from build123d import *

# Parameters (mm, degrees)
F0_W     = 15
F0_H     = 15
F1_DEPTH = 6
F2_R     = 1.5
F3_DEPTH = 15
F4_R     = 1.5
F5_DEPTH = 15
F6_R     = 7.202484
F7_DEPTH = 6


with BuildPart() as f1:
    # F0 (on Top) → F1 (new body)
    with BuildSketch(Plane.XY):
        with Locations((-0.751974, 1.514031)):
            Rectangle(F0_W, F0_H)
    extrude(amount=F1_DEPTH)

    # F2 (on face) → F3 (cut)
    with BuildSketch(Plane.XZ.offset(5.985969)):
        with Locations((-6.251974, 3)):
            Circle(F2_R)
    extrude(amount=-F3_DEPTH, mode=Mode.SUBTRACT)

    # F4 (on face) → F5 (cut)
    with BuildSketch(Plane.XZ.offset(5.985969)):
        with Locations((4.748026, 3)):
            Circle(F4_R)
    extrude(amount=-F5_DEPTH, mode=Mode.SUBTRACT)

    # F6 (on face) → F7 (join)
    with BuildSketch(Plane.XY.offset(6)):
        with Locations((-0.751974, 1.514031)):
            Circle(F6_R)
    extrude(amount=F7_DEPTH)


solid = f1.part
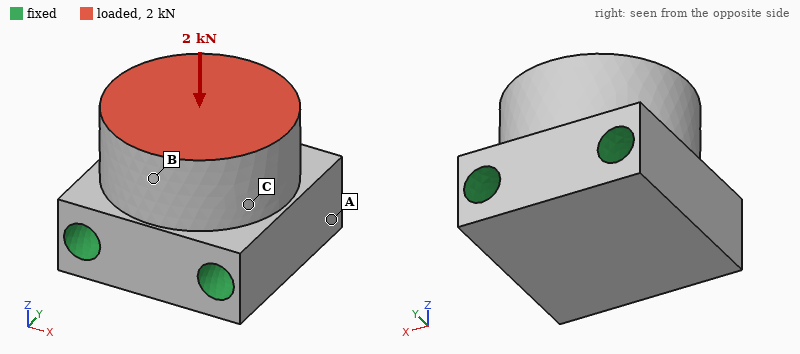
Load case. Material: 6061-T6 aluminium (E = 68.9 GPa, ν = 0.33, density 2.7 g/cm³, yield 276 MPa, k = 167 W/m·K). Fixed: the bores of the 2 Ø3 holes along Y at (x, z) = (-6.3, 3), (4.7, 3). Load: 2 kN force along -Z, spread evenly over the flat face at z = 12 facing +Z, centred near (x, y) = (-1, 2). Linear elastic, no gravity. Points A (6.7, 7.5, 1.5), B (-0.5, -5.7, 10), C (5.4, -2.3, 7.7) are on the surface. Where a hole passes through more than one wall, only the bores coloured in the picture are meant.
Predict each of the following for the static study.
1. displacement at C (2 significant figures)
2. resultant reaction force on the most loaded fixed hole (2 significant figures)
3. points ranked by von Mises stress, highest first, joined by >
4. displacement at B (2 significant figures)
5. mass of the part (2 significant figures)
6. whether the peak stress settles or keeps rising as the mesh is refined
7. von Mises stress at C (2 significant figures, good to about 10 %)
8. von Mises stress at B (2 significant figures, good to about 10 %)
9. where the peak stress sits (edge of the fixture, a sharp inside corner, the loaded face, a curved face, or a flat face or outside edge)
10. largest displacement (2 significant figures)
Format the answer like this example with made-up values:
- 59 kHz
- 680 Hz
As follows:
- 0.78 µm
- 1.0 kN
- C > B > A
- 1.5 µm
- 5.7 g
- keeps rising
- 16 MPa
- 11 MPa
- edge of the fixture
- 1.9 µm
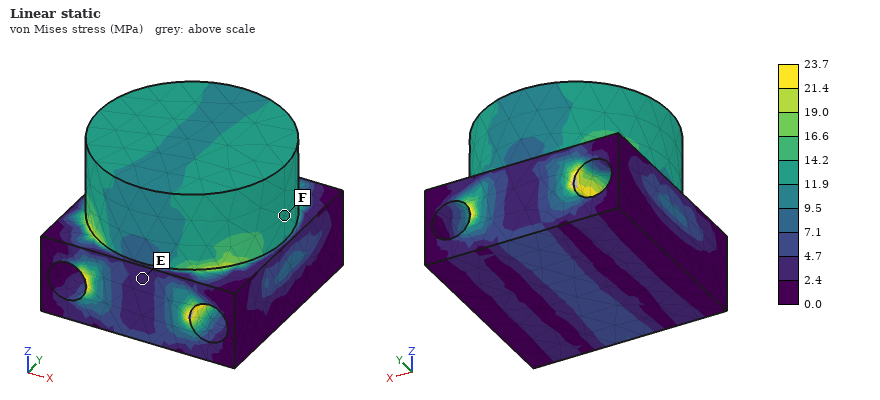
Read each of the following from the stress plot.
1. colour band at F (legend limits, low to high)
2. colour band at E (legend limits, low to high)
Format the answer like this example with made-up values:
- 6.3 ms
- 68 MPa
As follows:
- 11.9 to 14.2 MPa
- 2.4 to 4.7 MPa
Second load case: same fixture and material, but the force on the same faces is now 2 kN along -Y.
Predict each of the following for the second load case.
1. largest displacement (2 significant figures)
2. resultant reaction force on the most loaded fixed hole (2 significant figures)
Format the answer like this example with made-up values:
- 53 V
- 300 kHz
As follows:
- 9.6 µm
- 1.0 kN
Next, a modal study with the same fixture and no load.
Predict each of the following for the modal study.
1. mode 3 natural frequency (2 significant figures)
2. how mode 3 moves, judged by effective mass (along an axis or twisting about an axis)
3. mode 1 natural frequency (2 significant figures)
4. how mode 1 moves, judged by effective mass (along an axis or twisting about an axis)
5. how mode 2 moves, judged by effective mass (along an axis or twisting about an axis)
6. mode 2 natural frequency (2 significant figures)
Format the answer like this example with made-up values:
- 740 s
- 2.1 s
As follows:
- 100 kHz
- twisting about Z
- 70 kHz
- along Y
- along X
- 84 kHz
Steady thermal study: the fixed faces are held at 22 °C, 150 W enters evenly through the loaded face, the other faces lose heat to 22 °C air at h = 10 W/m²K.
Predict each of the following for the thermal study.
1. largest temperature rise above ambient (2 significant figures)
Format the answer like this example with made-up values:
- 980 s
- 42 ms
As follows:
- 47 K
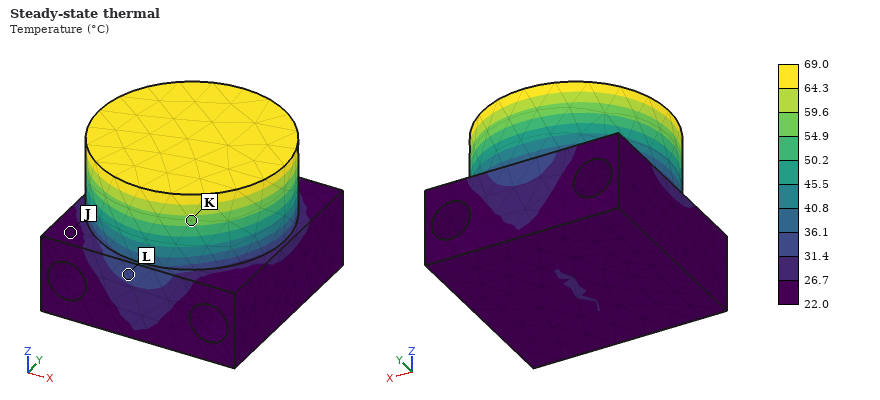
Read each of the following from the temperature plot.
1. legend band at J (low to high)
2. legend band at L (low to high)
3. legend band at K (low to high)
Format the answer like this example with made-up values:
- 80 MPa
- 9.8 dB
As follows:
- 22.0 to 26.7 °C
- 31.4 to 36.1 °C
- 54.9 to 59.6 °C
